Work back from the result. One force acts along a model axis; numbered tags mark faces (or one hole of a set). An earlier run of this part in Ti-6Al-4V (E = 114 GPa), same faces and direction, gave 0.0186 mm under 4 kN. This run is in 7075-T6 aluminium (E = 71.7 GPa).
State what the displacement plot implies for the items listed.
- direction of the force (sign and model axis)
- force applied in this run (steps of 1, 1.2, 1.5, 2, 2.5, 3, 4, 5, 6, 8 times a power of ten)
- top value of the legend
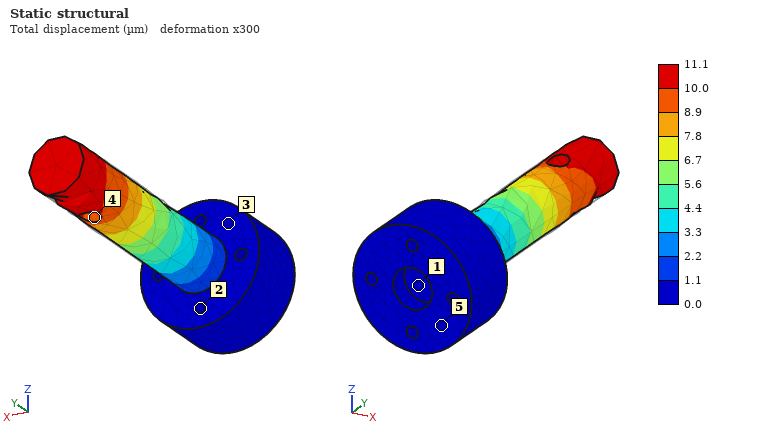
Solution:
+Y
1.5 kN
11.1 µm
